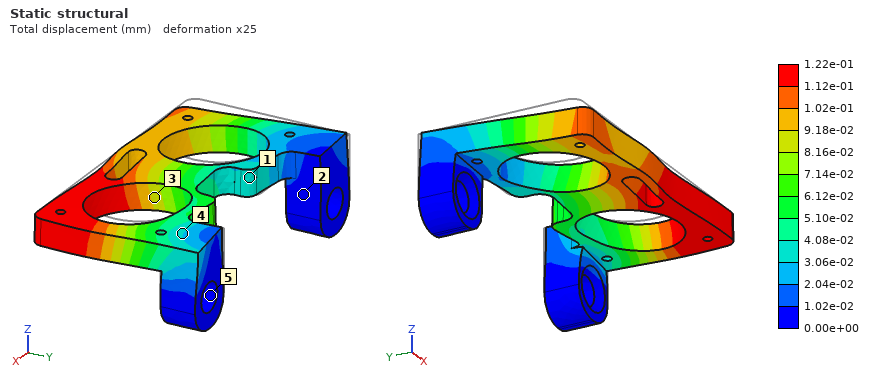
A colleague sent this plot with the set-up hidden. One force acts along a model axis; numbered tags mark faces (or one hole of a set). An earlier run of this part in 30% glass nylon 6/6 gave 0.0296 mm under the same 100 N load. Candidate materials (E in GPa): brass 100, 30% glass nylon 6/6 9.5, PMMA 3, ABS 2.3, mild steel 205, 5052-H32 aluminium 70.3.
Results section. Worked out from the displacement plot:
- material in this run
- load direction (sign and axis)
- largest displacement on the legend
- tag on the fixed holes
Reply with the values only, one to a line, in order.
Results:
ABS
+X
1.22e-01 mm
5
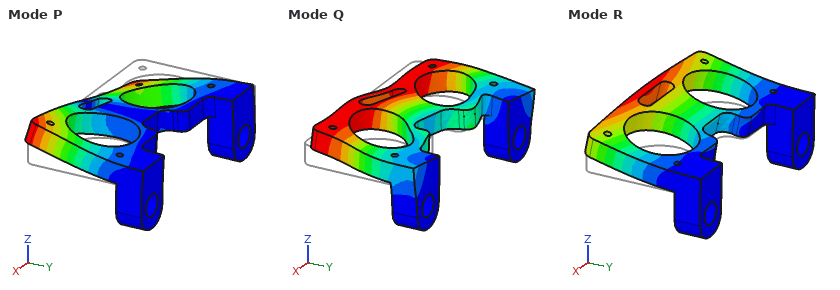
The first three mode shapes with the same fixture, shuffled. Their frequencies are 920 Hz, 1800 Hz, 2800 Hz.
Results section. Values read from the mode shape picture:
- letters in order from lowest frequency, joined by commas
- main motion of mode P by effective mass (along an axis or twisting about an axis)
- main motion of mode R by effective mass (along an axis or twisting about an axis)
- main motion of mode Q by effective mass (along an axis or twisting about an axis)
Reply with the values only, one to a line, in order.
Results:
R, P, Q
twisting about Y
along Z
along X
